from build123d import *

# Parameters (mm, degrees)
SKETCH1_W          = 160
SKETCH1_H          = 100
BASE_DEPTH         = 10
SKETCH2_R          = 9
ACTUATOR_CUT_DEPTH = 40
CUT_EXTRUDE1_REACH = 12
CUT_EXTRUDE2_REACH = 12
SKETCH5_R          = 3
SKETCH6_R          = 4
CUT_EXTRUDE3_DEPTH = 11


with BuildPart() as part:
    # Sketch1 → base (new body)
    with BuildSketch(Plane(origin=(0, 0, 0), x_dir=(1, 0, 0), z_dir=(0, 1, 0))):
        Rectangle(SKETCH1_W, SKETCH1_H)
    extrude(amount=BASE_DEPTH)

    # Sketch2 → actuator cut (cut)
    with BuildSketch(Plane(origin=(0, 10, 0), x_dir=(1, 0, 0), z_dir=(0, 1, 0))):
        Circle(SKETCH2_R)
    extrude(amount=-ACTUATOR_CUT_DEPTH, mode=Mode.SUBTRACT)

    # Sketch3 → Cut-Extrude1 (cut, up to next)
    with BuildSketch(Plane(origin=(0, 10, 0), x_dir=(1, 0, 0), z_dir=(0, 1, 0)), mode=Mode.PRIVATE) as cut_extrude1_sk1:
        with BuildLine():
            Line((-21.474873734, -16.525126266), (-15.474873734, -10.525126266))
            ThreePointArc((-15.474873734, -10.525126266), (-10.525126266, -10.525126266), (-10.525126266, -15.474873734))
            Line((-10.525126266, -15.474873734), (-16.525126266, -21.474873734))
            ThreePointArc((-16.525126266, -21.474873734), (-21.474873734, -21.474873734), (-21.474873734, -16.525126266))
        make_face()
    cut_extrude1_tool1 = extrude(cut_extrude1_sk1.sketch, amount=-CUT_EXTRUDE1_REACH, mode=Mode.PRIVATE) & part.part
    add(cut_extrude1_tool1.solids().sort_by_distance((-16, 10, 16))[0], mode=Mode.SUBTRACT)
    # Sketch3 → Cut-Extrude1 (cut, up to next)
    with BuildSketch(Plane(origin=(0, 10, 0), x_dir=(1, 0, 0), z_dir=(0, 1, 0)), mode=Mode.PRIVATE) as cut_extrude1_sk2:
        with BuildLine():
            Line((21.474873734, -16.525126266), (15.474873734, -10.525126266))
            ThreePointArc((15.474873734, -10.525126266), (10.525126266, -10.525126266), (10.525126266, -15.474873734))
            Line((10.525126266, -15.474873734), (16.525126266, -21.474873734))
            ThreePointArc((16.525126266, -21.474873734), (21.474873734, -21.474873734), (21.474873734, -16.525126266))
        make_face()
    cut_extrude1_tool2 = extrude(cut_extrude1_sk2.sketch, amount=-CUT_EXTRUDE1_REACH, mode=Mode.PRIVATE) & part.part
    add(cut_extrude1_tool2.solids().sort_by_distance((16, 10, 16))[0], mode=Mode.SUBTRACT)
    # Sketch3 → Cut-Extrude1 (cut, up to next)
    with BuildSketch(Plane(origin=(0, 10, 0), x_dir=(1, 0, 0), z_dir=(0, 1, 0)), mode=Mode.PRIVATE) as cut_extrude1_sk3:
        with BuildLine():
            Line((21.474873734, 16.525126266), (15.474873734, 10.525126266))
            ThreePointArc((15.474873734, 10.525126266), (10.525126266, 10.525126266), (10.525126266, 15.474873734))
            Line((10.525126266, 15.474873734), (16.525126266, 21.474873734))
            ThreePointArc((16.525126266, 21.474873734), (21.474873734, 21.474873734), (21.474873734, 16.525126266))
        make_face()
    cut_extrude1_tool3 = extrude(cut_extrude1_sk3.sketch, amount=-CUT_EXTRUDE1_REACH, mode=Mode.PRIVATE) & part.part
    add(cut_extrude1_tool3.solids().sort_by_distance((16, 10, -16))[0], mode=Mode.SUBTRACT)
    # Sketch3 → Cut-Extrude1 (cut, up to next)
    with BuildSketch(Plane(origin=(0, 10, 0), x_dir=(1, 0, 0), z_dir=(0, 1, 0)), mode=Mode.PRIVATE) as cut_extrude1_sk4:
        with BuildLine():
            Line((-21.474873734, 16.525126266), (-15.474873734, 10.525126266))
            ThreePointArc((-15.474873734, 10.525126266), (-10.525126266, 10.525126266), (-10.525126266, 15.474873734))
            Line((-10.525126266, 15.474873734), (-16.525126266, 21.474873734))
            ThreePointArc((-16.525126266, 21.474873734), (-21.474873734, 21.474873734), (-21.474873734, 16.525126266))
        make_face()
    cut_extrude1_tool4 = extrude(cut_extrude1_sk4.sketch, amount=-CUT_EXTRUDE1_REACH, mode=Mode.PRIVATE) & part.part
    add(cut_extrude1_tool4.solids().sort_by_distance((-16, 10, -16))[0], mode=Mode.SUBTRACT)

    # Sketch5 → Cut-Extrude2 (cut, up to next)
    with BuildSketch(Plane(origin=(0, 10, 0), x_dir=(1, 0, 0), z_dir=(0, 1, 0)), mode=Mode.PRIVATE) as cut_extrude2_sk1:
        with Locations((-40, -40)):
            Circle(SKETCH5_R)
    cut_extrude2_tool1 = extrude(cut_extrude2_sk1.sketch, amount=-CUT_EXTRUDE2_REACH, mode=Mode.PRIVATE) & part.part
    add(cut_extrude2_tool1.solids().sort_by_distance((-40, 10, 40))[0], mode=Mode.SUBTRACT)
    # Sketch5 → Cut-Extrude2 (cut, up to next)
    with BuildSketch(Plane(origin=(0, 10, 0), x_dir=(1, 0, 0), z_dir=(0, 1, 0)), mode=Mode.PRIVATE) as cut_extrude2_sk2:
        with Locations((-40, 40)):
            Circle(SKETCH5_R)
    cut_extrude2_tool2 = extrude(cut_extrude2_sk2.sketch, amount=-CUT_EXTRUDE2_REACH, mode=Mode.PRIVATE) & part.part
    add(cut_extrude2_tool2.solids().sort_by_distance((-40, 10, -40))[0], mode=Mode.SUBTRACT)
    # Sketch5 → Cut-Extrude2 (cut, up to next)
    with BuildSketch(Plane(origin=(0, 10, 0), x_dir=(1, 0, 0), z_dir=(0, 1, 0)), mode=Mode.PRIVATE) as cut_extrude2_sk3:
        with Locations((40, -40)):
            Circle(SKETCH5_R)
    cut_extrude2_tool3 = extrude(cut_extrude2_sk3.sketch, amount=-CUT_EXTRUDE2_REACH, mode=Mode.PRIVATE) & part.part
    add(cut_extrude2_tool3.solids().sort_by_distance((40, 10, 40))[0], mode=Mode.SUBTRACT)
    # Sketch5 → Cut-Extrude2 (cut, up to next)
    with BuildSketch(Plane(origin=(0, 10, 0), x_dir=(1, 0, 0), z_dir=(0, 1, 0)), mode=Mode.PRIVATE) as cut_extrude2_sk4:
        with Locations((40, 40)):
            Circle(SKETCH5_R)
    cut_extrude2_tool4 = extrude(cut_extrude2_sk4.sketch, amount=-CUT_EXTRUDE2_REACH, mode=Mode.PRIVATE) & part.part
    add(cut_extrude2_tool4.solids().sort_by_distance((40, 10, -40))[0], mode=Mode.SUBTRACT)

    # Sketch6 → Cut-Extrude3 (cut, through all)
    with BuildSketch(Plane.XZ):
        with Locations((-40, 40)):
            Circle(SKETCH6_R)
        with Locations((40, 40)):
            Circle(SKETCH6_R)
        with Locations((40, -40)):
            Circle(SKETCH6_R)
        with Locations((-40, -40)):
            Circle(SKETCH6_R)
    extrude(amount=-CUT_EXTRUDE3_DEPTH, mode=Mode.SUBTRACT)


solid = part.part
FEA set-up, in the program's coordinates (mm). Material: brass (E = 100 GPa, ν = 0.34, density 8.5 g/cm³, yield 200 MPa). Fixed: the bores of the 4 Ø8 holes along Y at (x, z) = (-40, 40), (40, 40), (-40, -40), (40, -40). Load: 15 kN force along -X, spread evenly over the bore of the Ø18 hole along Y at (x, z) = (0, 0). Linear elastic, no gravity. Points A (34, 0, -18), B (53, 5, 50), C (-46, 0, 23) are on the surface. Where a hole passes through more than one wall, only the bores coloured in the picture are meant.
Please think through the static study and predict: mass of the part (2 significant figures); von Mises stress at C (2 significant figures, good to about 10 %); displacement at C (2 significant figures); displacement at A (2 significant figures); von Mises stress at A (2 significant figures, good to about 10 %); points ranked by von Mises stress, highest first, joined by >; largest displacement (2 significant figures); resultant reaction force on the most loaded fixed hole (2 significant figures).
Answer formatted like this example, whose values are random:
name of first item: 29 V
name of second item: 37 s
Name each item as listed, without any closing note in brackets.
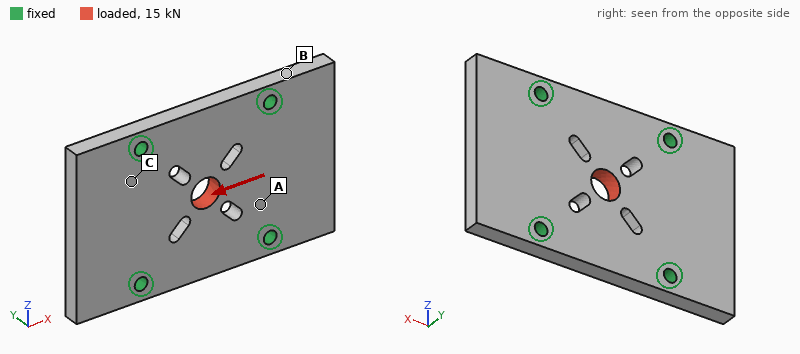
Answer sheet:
mass of the part: 1.3 kg
von Mises stress at C: 8.5 MPa
displacement at C: 3.2 µm
displacement at A: 4.2 µm
von Mises stress at A: 12 MPa
points ranked by von Mises stress, highest first, joined by >: A > C > B
largest displacement: 11 µm
resultant reaction force on the most loaded fixed hole: 3.9 kN
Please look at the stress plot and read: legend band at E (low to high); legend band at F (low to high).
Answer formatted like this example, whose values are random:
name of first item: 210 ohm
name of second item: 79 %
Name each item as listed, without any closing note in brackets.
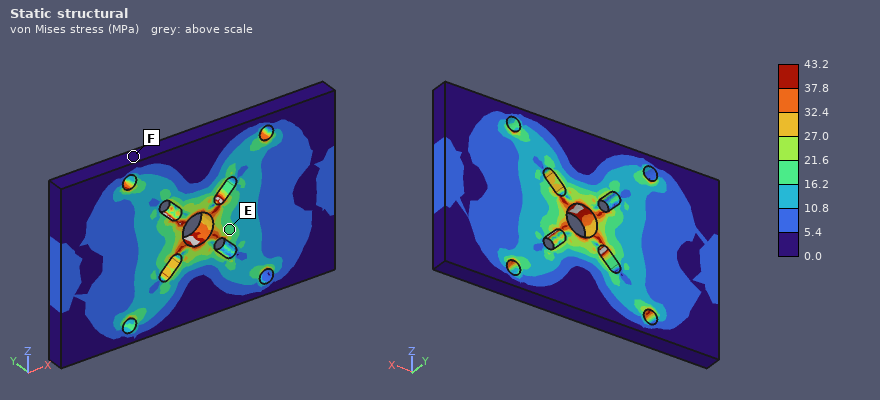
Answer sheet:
legend band at E: 16.2 to 21.6 MPa
legend band at F: 0.0 to 5.4 MPa
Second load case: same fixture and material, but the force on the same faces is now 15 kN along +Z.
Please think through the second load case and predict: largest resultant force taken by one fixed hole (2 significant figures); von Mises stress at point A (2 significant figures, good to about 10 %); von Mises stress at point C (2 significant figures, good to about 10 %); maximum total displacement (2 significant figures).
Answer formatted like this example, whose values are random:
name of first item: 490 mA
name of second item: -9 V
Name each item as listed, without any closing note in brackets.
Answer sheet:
largest resultant force taken by one fixed hole: 4.3 kN
von Mises stress at point A: 15 MPa
von Mises stress at point C: 6.2 MPa
maximum total displacement: 14 µm
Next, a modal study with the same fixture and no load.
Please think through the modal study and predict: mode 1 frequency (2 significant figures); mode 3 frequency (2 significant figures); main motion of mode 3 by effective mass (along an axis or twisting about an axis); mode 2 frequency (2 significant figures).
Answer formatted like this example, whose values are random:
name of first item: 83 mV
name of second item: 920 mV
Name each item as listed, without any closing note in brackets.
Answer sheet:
mode 1 frequency: 2600 Hz
mode 3 frequency: 3700 Hz
main motion of mode 3 by effective mass: along Y
mode 2 frequency: 2600 Hz
